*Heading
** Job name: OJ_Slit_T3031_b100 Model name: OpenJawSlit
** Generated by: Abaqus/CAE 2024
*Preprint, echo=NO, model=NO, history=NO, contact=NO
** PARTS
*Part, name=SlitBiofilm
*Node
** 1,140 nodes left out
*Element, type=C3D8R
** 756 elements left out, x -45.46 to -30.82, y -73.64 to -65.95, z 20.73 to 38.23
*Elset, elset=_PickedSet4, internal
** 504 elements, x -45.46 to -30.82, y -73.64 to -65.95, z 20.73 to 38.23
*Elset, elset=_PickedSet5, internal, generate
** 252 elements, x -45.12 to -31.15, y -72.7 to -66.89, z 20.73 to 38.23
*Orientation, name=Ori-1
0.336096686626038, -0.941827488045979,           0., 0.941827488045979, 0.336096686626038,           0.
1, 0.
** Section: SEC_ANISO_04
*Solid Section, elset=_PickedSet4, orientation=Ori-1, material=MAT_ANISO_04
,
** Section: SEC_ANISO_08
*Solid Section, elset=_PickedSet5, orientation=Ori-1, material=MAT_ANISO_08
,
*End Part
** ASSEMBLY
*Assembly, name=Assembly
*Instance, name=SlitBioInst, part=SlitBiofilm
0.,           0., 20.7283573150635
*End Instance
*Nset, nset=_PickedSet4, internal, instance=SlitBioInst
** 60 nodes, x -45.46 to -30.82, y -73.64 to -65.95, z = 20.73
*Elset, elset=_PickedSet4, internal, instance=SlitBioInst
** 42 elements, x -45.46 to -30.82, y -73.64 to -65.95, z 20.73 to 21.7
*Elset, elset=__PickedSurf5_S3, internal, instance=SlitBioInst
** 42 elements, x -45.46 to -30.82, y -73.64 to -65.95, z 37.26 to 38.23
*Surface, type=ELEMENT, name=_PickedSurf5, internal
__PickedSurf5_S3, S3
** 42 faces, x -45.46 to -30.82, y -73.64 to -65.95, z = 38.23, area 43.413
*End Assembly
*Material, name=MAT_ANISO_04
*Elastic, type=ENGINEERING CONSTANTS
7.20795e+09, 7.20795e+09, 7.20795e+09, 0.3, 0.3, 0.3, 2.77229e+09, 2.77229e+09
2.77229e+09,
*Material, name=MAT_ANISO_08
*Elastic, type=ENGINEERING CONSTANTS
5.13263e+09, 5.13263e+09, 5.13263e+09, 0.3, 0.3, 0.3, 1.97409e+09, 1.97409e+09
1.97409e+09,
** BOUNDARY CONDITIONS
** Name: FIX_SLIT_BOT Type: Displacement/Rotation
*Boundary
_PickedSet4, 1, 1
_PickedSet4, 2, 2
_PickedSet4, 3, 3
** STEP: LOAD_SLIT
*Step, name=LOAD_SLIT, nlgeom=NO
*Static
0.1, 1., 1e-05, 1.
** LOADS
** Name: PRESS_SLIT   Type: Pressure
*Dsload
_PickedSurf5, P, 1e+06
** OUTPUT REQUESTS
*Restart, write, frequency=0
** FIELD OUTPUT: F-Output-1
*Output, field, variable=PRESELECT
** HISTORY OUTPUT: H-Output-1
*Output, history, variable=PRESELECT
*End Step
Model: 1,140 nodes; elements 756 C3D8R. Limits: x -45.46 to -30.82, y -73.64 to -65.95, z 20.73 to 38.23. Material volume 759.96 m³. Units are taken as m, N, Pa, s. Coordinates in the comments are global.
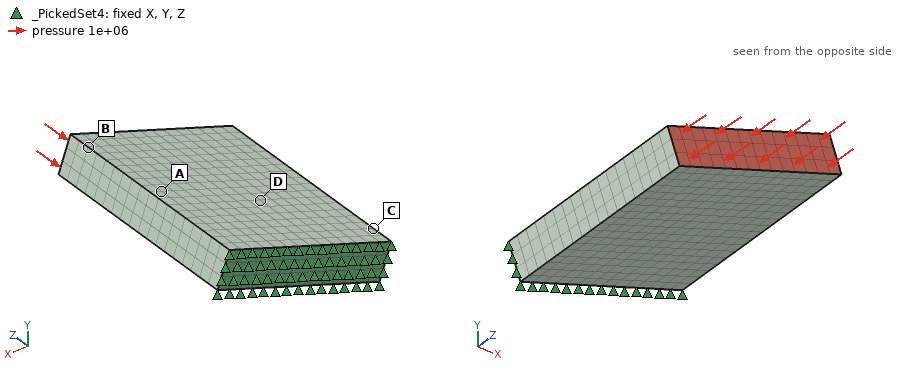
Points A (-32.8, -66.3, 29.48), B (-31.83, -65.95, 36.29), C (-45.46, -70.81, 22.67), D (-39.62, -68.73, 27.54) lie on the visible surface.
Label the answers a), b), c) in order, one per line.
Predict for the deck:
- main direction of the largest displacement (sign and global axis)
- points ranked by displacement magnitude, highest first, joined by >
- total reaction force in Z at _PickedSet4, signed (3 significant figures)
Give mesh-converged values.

a) -Z
b) B > A > D > C
c) 4.34e+07 N
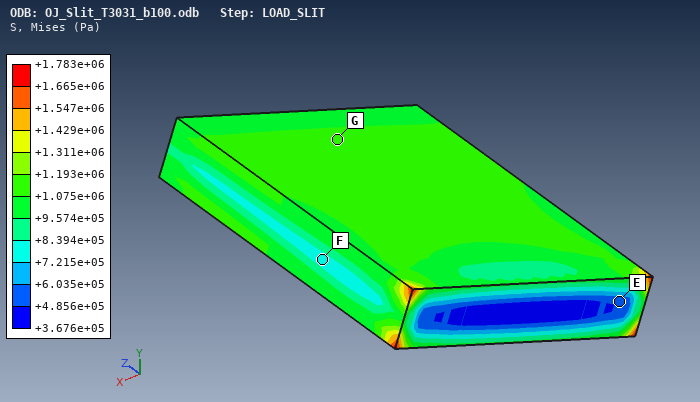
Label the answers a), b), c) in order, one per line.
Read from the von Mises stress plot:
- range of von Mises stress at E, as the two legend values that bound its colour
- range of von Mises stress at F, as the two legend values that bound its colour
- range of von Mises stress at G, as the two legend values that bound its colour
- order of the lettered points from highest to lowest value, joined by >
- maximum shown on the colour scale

a) +4.856e+05 to +6.035e+05 Pa
b) +7.215e+05 to +8.394e+05 Pa
c) +1.075e+06 to +1.193e+06 Pa
d) G > F > E
e) +1.783e+06 Pa
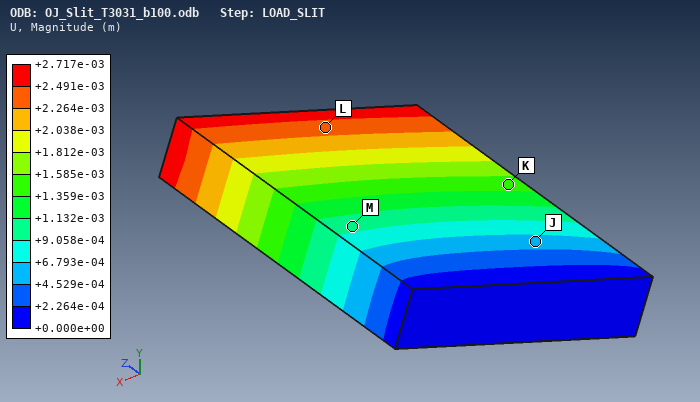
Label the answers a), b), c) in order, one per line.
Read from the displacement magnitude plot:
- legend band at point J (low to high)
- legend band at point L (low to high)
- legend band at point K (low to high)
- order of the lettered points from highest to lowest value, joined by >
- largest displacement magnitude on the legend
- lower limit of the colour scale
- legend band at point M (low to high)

a) +4.529e-04 to +6.793e-04 m
b) +2.264e-03 to +2.491e-03 m
c) +1.359e-03 to +1.585e-03 m
d) L > K > M > J
e) +2.717e-03 m
f) +0.000e+00 m
g) +9.058e-04 to +1.132e-03 m
